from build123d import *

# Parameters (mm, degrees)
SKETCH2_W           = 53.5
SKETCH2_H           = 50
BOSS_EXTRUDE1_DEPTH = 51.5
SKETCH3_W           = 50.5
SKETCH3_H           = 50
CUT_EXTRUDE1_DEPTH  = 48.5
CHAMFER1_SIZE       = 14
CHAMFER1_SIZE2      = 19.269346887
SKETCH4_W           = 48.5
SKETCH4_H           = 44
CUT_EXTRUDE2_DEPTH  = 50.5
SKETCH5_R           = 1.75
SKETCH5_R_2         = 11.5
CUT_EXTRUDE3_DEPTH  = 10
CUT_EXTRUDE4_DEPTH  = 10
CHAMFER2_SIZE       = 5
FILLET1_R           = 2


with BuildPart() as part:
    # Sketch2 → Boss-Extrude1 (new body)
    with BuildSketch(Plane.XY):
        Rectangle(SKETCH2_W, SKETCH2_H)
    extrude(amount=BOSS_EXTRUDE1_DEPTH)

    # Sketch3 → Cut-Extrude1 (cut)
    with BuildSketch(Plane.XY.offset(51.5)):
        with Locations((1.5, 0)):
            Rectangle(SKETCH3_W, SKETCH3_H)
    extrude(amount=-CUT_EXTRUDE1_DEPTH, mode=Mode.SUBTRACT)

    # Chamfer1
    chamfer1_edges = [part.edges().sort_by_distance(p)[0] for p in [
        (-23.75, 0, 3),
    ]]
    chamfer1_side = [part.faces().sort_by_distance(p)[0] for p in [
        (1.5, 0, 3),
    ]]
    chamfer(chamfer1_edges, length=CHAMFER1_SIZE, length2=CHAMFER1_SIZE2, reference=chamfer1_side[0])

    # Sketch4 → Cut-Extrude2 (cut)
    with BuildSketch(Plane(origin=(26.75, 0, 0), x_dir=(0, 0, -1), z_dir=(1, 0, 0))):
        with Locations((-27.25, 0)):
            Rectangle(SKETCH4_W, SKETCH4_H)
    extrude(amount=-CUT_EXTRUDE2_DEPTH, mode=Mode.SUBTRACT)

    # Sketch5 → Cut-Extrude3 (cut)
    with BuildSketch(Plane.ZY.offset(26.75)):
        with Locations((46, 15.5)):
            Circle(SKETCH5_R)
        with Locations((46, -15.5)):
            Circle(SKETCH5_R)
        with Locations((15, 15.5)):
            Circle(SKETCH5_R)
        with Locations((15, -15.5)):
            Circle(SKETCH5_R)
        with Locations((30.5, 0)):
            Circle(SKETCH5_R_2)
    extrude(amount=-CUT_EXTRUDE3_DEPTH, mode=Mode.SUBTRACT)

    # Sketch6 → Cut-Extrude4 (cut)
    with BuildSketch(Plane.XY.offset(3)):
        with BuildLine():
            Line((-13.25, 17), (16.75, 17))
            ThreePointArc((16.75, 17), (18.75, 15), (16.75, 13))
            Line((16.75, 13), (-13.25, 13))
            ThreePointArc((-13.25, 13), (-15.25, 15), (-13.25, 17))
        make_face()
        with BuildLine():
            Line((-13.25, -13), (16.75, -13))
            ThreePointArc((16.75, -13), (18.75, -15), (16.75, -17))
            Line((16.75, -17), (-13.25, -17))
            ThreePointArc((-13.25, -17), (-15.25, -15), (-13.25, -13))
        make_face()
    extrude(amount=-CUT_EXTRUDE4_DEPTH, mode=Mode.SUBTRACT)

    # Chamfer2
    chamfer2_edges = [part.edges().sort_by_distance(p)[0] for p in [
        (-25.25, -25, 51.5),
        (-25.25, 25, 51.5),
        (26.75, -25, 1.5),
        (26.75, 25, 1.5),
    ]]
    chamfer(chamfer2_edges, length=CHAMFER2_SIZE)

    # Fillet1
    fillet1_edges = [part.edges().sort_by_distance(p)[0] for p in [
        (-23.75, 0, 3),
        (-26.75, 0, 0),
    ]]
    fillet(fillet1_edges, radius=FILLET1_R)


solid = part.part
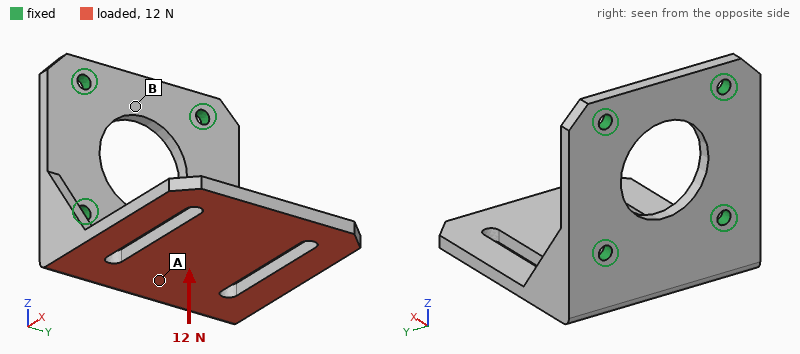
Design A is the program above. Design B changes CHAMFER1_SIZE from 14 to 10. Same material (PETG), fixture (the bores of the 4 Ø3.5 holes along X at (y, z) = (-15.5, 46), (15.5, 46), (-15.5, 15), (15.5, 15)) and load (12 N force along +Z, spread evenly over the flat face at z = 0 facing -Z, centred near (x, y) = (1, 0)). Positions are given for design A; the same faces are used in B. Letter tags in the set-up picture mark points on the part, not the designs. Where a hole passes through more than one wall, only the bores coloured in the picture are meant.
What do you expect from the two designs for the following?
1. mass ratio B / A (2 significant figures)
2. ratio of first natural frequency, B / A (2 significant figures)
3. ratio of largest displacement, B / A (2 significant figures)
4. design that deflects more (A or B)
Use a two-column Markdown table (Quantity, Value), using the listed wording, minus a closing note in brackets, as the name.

| Quantity | Value |
|---|---|
| mass ratio B / A | 0.98 |
| ratio of first natural frequency, B / A | 0.92 |
| ratio of largest displacement, B / A | 1.2 |
| design that deflects more | B |
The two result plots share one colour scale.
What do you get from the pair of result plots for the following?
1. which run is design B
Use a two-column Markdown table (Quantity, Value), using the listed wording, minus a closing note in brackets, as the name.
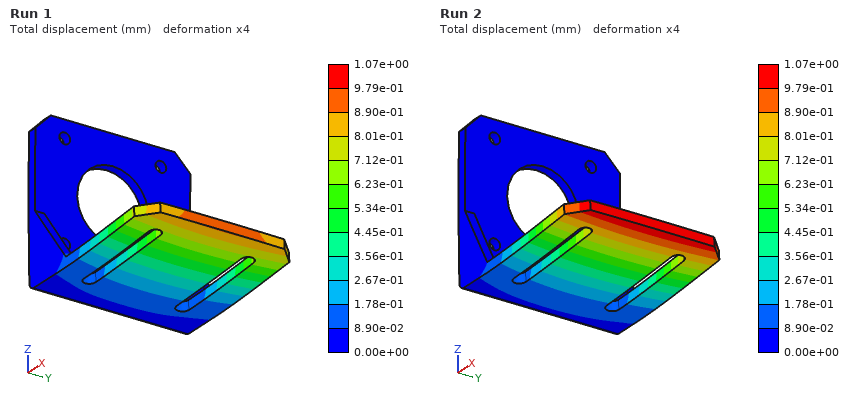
| Quantity | Value |
|---|---|
| which run is design B | Run 2 |
